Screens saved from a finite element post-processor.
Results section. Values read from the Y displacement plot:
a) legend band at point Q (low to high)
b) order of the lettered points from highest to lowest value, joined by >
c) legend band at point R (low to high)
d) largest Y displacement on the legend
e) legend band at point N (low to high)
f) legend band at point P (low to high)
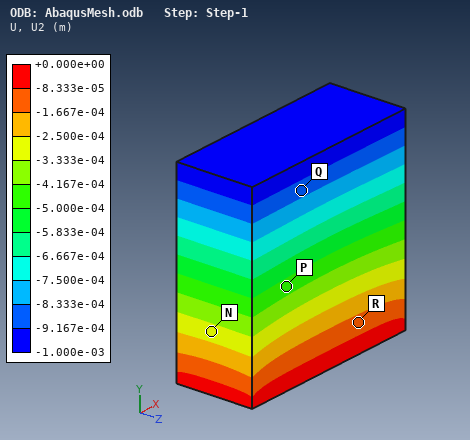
-9.167e-04 to -8.333e-04 m
R > N > P > Q
-1.667e-04 to -8.333e-05 m
+0.000e+00 m
-3.333e-04 to -2.500e-04 m
-5.000e-04 to -4.167e-04 m
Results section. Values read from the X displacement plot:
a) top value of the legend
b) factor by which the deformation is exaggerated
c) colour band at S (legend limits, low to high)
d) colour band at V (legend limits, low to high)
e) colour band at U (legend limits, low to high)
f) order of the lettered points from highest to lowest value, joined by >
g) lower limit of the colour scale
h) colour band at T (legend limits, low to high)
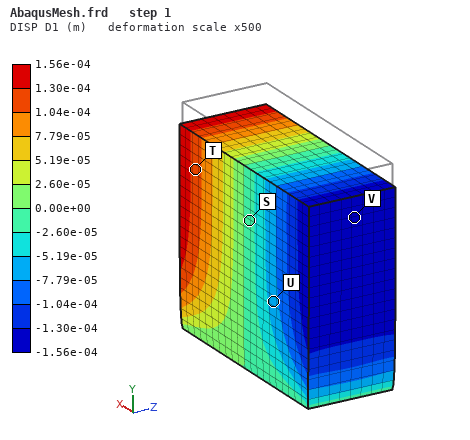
1.56e-04 m
500
-2.60e-05 to 0.00e+00 m
-1.56e-04 to -1.30e-04 m
-7.79e-05 to -5.19e-05 m
T > S > U > V
-1.56e-04 m
1.04e-04 to 1.30e-04 m
